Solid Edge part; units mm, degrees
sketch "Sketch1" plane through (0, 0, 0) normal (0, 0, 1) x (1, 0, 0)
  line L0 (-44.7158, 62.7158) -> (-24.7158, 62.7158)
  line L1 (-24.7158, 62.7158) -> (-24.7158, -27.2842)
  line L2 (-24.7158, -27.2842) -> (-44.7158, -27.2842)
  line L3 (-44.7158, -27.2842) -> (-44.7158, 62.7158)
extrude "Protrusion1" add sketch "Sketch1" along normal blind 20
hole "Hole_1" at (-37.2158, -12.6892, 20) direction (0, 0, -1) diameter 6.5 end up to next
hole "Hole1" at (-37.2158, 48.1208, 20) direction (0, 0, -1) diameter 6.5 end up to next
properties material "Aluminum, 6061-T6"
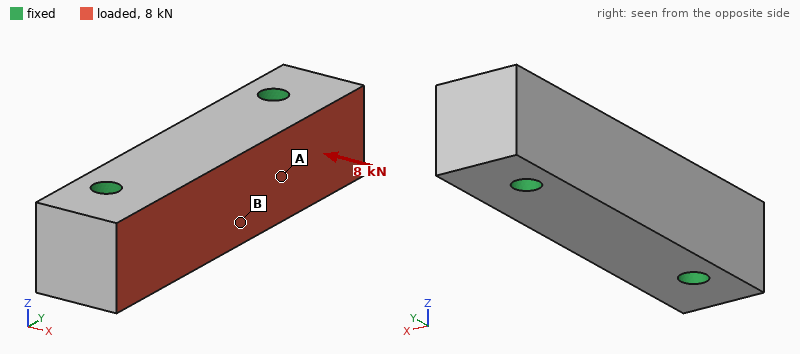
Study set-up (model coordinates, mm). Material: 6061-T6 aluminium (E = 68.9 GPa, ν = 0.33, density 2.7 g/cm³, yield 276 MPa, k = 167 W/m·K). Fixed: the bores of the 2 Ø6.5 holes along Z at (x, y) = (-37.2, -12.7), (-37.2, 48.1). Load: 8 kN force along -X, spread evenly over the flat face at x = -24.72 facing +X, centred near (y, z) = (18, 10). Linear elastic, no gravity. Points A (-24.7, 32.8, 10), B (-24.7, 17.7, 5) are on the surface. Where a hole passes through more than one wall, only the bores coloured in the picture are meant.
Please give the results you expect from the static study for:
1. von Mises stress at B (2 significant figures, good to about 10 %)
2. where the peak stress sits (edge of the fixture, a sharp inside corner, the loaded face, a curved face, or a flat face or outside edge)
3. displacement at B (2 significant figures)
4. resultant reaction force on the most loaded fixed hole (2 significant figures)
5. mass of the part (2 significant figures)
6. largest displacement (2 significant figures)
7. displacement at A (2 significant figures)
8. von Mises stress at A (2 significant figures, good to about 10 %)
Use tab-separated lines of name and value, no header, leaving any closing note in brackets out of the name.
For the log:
von Mises stress at B	14 MPa
where the peak stress sits	edge of the fixture
displacement at B	9.2 µm
resultant reaction force on the most loaded fixed hole	4.1 kN
mass of the part	94 g
largest displacement	9.5 µm
displacement at A	6.8 µm
von Mises stress at A	6.8 MPa
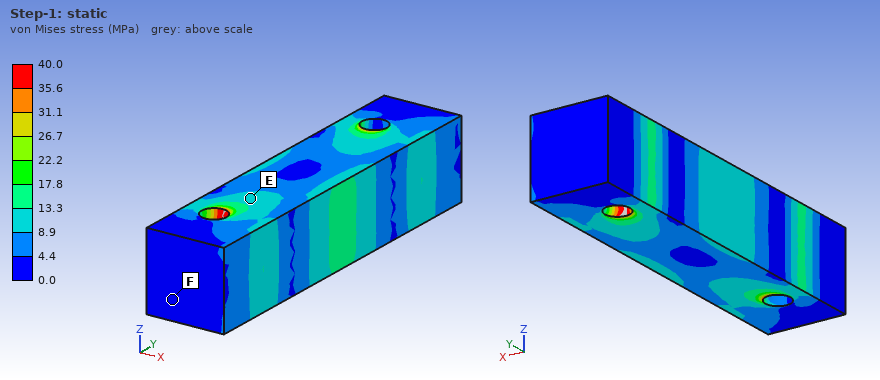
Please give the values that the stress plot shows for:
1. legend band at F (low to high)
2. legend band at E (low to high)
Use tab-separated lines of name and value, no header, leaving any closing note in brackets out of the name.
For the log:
legend band at F	0.0 to 4.4 MPa
legend band at E	8.9 to 13.3 MPa
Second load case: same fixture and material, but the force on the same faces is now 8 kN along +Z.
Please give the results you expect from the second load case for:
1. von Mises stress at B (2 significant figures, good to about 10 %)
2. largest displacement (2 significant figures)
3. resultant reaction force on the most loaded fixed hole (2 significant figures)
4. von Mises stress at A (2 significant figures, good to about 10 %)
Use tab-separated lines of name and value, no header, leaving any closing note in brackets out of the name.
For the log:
von Mises stress at B	9.3 MPa
largest displacement	20 µm
resultant reaction force on the most loaded fixed hole	4.0 kN
von Mises stress at A	24 MPa
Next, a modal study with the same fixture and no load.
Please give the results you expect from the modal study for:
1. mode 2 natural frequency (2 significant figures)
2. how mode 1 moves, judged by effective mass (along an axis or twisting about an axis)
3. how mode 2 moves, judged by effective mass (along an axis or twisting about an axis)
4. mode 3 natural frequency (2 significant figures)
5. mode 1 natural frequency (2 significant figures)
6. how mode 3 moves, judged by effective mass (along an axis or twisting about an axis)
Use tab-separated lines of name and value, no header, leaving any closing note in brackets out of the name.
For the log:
mode 2 natural frequency	18 kHz
how mode 1 moves, judged by effective mass	along X
how mode 2 moves, judged by effective mass	along Z
mode 3 natural frequency	24 kHz
mode 1 natural frequency	16 kHz
how mode 3 moves, judged by effective mass	twisting about Y
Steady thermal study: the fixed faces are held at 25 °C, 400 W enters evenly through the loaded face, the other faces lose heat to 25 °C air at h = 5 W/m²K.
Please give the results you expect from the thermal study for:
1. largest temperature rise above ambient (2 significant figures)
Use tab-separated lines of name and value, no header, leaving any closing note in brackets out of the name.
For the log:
largest temperature rise above ambient	42 K
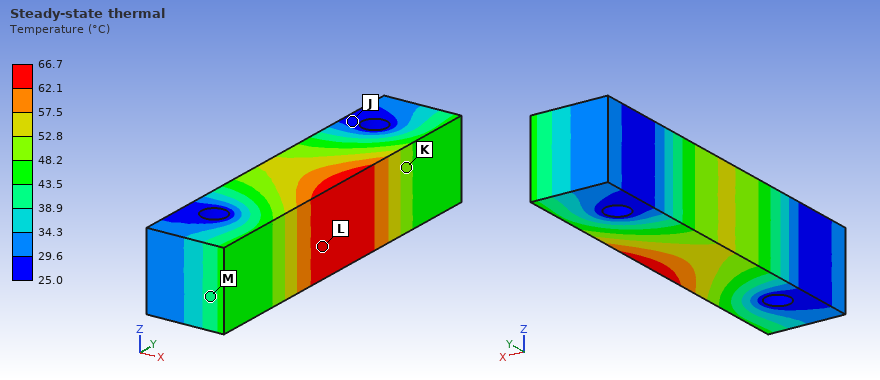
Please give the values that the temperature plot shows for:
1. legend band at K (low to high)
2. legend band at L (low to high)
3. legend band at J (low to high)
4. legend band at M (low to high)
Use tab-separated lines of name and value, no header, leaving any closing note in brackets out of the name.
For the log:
legend band at K	48.2 to 52.8 °C
legend band at L	62.1 to 66.7 °C
legend band at J	25.0 to 29.6 °C
legend band at M	38.9 to 43.5 °C
